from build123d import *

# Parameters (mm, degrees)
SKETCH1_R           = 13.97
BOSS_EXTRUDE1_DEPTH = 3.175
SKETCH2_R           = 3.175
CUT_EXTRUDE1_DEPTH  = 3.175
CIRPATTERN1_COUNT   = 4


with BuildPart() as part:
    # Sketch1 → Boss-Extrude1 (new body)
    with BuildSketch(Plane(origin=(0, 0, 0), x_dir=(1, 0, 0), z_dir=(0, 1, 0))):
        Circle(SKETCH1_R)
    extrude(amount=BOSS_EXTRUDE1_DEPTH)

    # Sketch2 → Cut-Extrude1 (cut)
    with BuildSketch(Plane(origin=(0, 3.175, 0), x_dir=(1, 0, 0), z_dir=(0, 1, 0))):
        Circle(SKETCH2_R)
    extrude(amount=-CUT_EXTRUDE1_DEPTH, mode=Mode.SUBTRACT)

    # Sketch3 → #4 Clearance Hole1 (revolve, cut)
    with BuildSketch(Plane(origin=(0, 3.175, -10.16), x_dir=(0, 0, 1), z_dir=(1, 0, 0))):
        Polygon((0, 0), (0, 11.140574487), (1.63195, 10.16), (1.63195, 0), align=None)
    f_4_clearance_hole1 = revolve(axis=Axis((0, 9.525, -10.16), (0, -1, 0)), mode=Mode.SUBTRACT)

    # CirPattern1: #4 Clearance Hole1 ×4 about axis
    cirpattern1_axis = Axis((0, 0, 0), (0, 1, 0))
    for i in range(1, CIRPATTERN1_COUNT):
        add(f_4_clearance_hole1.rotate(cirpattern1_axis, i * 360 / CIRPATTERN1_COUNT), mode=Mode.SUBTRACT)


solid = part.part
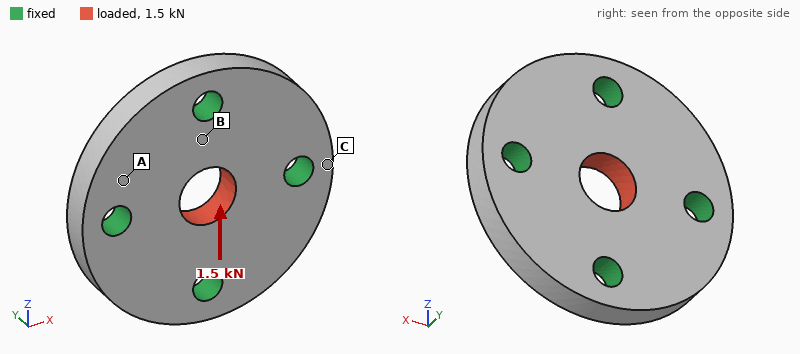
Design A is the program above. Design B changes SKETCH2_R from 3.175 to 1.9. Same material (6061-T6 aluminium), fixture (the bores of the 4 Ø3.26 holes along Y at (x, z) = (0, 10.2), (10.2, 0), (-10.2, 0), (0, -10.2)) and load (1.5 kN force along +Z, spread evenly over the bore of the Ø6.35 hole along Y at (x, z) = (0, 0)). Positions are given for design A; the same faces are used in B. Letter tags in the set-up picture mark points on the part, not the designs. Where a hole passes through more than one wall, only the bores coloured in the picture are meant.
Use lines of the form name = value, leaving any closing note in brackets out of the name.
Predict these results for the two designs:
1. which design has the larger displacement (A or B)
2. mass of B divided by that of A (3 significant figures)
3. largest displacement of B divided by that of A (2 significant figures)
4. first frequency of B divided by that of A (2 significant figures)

which design has the larger displacement = B
mass of B divided by that of A = 1.04
largest displacement of B divided by that of A = 1.3
first frequency of B divided by that of A = 1.0
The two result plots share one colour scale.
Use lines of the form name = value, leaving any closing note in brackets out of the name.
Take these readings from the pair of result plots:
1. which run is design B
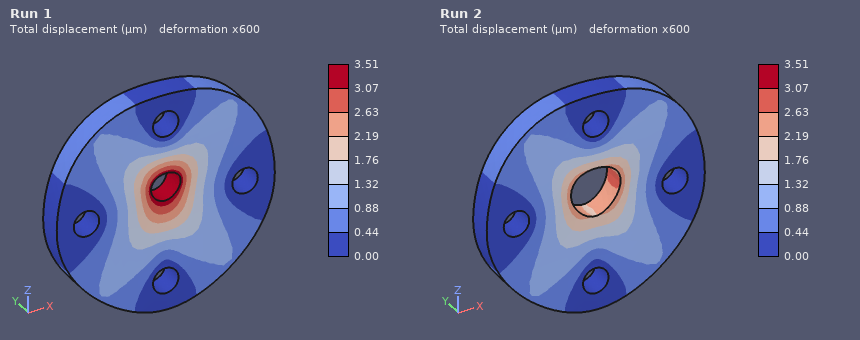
which run is design B = Run 1
